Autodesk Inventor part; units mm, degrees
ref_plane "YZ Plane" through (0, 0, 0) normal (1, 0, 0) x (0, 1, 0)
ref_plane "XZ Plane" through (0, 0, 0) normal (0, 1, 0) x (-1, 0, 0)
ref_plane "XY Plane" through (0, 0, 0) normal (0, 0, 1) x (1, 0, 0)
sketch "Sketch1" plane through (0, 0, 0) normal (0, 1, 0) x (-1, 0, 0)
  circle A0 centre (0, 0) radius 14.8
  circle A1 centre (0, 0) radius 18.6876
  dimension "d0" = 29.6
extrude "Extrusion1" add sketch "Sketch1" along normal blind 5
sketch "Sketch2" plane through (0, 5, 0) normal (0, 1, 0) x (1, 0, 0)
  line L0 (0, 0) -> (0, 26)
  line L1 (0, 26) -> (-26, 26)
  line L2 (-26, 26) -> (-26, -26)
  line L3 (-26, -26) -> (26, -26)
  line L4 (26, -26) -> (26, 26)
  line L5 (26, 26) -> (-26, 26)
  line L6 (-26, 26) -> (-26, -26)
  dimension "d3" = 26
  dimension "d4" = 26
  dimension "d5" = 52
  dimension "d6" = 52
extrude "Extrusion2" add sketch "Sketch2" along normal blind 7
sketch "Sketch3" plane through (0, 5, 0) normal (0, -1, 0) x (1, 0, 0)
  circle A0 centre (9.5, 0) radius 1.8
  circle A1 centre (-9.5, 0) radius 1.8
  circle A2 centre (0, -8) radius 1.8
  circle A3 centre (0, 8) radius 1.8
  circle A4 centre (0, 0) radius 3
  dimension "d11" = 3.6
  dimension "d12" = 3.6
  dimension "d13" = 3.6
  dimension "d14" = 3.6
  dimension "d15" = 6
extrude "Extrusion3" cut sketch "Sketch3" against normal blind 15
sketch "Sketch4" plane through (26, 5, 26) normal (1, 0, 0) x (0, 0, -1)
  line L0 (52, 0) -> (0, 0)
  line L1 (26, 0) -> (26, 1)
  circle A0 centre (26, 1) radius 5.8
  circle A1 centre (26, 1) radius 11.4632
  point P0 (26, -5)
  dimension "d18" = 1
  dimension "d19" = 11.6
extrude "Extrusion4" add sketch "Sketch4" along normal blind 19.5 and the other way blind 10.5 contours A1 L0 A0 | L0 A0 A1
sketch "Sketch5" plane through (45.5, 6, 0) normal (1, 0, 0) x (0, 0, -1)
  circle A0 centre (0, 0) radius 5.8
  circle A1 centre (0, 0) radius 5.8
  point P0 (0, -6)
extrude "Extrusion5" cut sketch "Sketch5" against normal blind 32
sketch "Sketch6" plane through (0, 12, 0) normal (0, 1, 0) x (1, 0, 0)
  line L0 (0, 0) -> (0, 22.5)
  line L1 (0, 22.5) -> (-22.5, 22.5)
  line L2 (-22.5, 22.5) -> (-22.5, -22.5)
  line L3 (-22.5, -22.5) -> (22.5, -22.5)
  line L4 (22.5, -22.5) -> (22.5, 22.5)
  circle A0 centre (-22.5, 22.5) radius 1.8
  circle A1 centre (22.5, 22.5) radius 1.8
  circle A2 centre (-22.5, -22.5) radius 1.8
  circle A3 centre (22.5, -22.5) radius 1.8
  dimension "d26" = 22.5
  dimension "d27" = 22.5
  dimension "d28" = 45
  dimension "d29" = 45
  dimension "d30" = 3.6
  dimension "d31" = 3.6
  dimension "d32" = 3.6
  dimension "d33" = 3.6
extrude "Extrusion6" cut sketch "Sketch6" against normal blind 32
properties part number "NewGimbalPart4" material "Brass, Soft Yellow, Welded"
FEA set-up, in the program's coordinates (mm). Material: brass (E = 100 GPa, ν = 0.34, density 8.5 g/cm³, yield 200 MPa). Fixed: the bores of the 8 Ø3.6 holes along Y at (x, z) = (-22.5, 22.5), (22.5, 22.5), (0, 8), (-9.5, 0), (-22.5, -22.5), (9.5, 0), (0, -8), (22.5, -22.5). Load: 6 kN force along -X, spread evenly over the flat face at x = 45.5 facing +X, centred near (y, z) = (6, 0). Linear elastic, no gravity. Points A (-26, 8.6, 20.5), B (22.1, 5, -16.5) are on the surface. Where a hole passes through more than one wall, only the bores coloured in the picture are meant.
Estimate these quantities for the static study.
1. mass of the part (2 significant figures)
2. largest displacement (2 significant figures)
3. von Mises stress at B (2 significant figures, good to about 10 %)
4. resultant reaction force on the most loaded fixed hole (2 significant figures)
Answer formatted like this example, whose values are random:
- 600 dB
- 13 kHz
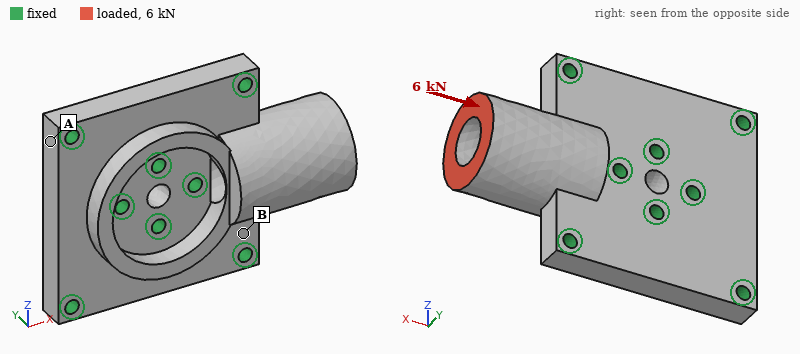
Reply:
- 230 g
- 27 µm
- 28 MPa
- 1.3 kN
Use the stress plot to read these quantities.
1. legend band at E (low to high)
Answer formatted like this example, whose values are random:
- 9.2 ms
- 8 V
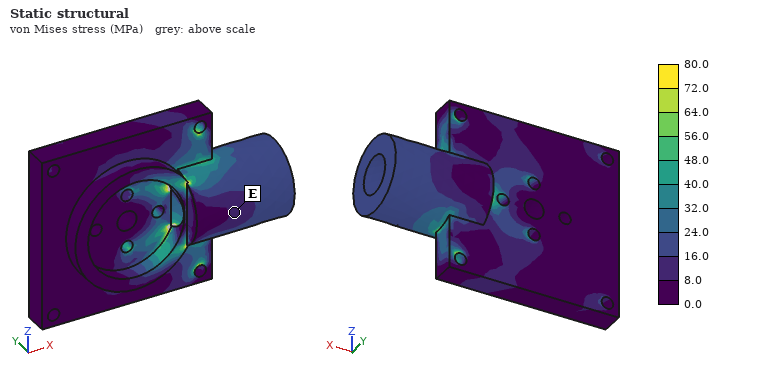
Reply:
- 8.0 to 16.0 MPa
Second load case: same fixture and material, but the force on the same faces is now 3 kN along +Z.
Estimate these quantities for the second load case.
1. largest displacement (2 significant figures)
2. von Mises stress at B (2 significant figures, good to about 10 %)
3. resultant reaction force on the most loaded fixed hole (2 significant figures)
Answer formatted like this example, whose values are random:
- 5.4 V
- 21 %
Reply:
- 38 µm
- 40 MPa
- 1.6 kN
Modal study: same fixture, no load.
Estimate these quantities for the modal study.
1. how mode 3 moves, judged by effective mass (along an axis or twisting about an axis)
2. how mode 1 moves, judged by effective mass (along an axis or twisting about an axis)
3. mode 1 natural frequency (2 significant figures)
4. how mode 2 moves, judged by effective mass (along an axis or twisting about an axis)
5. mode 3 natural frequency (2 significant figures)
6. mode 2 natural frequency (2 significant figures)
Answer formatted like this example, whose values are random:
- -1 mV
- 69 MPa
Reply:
- twisting about X
- along Y
- 4200 Hz
- along Z
- 14 kHz
- 9800 Hz
